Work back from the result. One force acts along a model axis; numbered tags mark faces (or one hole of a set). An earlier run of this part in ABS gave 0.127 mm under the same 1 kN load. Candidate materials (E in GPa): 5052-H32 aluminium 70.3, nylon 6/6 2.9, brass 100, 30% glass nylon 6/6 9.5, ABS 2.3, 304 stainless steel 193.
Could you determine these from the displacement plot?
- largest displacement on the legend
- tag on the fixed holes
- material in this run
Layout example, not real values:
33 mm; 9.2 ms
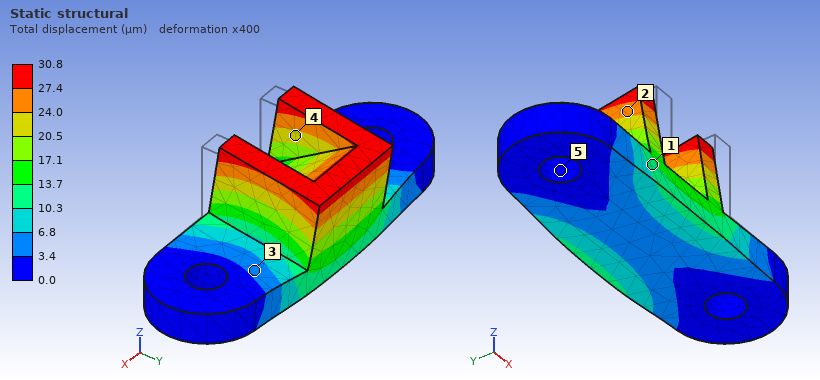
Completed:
30.8 µm; 5; 30% glass nylon 6/6
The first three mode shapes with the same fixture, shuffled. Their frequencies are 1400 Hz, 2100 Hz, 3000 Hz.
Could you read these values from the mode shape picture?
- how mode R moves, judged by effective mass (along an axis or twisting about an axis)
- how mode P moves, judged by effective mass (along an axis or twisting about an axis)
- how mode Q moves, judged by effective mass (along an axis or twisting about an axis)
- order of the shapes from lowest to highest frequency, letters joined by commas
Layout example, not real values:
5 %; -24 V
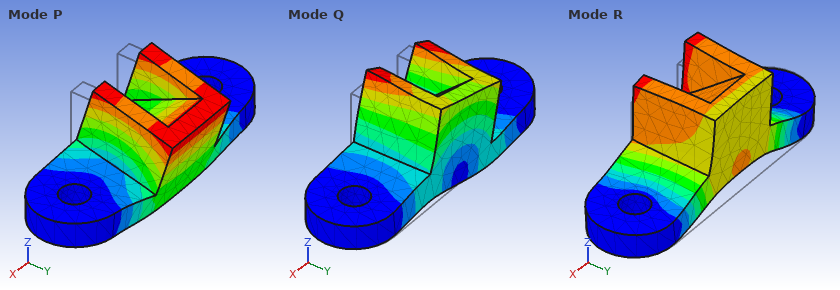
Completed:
along Z; along Y; along X; P, R, Q
